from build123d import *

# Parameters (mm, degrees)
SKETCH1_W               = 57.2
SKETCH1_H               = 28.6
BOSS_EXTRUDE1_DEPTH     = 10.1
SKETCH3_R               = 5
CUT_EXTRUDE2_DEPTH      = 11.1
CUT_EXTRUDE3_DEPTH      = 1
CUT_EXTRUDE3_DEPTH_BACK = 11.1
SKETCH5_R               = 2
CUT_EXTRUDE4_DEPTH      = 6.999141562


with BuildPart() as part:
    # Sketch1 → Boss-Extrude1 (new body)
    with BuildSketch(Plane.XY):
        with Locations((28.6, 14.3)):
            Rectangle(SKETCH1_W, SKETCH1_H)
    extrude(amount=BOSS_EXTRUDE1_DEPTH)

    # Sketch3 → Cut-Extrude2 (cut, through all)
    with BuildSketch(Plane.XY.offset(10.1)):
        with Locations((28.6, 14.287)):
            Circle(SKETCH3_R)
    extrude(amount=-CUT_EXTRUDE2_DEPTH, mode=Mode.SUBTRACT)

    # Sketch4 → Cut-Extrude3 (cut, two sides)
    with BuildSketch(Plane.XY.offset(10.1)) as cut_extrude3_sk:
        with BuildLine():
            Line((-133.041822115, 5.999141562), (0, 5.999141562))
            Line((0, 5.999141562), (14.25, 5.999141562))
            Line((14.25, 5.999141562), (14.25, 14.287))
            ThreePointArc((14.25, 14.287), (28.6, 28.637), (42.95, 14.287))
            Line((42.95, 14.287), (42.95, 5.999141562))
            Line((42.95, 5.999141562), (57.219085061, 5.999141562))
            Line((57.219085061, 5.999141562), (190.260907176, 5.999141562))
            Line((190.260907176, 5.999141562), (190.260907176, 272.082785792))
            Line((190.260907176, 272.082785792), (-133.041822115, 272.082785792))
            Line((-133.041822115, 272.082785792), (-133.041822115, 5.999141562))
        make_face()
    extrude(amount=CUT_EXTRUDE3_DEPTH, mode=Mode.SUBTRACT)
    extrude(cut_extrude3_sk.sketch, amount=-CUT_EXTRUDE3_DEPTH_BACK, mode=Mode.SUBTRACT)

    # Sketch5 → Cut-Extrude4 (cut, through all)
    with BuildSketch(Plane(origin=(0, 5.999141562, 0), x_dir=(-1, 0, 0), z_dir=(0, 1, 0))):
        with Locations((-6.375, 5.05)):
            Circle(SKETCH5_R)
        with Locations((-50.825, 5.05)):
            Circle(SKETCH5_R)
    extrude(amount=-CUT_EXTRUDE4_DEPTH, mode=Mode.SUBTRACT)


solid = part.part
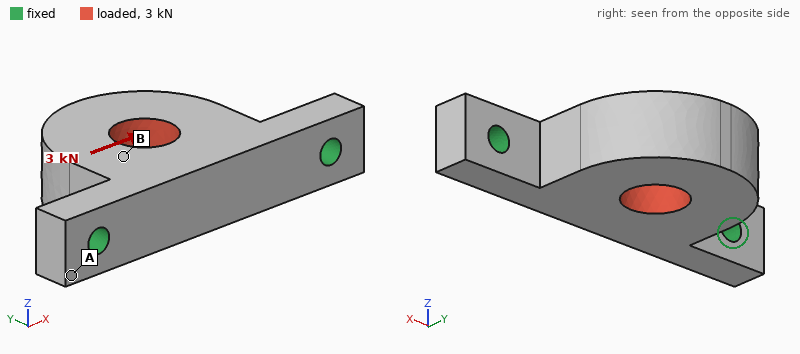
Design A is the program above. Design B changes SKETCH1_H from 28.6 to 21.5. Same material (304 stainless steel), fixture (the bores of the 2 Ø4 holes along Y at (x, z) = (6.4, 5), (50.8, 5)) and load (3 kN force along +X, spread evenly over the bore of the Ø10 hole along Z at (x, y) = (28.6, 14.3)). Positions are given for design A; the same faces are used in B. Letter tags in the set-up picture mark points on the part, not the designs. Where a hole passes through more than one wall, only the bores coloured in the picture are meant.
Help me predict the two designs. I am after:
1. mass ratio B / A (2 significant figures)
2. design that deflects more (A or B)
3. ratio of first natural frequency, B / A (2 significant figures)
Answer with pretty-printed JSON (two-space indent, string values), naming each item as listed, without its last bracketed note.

{
  "mass ratio B / A": "0.70",
  "design that deflects more": "B",
  "ratio of first natural frequency, B / A": "0.52"
}
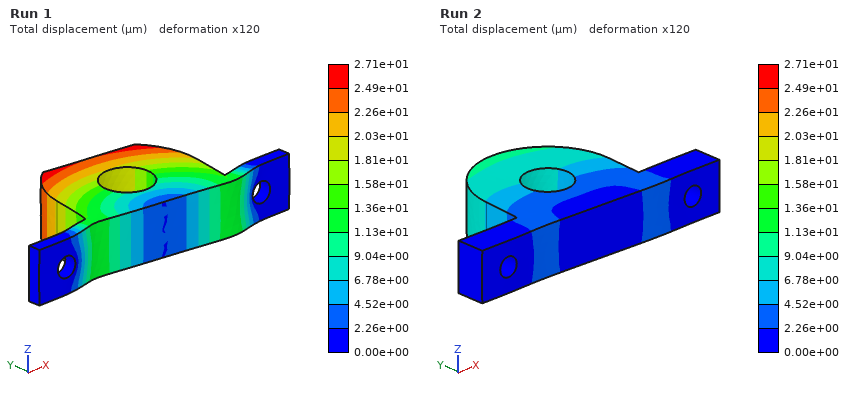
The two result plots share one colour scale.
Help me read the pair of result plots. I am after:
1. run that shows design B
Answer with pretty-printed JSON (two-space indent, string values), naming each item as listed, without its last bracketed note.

{
  "run that shows design B": "Run 1"
}
